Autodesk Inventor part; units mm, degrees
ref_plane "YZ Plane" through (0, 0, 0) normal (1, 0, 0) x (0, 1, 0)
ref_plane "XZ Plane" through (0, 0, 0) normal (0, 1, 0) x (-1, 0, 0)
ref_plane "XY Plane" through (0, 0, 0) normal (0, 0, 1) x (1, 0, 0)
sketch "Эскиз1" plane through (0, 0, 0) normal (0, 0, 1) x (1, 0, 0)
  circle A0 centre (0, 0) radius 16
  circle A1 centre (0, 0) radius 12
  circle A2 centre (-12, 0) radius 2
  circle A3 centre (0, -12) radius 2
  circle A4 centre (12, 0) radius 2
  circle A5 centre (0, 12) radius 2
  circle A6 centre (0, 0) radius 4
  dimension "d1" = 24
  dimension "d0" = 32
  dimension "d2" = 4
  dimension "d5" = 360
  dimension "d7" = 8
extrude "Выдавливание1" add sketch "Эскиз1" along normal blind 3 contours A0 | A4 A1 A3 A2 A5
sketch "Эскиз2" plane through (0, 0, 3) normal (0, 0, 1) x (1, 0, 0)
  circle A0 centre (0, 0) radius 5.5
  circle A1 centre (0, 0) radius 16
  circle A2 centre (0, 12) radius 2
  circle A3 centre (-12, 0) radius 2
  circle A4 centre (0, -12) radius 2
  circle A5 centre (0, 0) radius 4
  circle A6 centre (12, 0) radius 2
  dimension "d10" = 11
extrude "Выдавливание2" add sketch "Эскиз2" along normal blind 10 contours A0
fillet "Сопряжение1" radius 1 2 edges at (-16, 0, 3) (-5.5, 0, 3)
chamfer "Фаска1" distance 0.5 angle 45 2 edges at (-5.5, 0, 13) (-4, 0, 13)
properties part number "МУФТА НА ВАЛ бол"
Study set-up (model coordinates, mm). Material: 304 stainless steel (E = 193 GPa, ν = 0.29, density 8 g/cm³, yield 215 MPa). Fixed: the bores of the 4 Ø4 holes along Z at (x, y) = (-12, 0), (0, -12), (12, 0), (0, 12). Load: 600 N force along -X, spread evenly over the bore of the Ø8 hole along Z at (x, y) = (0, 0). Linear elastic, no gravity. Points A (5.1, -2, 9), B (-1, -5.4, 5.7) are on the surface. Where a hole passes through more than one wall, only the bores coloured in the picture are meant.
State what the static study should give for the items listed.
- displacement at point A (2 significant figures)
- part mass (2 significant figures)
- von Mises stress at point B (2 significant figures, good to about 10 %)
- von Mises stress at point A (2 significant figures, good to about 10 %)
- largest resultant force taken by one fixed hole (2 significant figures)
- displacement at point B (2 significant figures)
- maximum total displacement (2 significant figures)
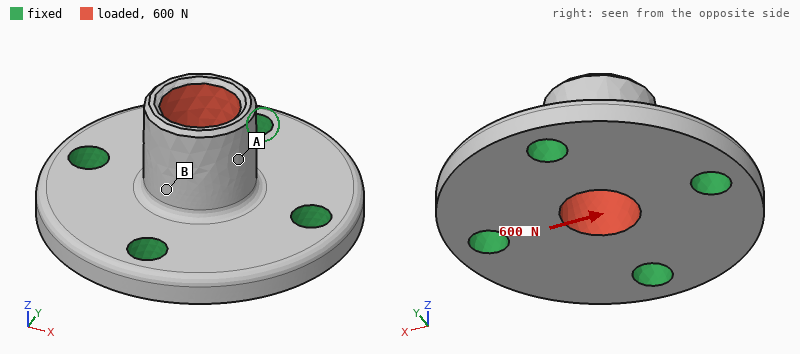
2.9 µm
20 g
16 MPa
6.5 MPa
250 N
1.4 µm
4.0 µm
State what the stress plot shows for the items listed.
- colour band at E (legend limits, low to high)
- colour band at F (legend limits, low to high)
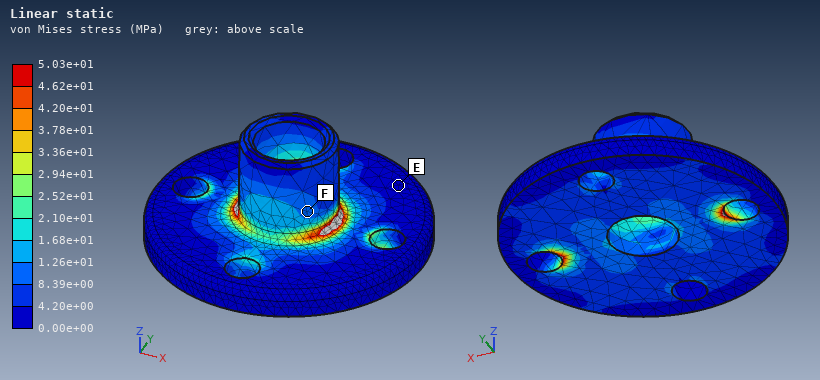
0.00e+00 to 4.20e+00 MPa
8.39e+00 to 1.26e+01 MPa
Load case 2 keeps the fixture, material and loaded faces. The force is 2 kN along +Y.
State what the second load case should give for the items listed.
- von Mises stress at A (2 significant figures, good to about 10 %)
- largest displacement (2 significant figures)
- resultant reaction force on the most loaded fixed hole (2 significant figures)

36 MPa
13 µm
830 N
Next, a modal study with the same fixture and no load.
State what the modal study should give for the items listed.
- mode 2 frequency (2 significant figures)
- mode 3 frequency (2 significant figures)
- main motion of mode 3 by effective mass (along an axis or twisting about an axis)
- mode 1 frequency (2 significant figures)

31 kHz
38 kHz
along Z
31 kHz
